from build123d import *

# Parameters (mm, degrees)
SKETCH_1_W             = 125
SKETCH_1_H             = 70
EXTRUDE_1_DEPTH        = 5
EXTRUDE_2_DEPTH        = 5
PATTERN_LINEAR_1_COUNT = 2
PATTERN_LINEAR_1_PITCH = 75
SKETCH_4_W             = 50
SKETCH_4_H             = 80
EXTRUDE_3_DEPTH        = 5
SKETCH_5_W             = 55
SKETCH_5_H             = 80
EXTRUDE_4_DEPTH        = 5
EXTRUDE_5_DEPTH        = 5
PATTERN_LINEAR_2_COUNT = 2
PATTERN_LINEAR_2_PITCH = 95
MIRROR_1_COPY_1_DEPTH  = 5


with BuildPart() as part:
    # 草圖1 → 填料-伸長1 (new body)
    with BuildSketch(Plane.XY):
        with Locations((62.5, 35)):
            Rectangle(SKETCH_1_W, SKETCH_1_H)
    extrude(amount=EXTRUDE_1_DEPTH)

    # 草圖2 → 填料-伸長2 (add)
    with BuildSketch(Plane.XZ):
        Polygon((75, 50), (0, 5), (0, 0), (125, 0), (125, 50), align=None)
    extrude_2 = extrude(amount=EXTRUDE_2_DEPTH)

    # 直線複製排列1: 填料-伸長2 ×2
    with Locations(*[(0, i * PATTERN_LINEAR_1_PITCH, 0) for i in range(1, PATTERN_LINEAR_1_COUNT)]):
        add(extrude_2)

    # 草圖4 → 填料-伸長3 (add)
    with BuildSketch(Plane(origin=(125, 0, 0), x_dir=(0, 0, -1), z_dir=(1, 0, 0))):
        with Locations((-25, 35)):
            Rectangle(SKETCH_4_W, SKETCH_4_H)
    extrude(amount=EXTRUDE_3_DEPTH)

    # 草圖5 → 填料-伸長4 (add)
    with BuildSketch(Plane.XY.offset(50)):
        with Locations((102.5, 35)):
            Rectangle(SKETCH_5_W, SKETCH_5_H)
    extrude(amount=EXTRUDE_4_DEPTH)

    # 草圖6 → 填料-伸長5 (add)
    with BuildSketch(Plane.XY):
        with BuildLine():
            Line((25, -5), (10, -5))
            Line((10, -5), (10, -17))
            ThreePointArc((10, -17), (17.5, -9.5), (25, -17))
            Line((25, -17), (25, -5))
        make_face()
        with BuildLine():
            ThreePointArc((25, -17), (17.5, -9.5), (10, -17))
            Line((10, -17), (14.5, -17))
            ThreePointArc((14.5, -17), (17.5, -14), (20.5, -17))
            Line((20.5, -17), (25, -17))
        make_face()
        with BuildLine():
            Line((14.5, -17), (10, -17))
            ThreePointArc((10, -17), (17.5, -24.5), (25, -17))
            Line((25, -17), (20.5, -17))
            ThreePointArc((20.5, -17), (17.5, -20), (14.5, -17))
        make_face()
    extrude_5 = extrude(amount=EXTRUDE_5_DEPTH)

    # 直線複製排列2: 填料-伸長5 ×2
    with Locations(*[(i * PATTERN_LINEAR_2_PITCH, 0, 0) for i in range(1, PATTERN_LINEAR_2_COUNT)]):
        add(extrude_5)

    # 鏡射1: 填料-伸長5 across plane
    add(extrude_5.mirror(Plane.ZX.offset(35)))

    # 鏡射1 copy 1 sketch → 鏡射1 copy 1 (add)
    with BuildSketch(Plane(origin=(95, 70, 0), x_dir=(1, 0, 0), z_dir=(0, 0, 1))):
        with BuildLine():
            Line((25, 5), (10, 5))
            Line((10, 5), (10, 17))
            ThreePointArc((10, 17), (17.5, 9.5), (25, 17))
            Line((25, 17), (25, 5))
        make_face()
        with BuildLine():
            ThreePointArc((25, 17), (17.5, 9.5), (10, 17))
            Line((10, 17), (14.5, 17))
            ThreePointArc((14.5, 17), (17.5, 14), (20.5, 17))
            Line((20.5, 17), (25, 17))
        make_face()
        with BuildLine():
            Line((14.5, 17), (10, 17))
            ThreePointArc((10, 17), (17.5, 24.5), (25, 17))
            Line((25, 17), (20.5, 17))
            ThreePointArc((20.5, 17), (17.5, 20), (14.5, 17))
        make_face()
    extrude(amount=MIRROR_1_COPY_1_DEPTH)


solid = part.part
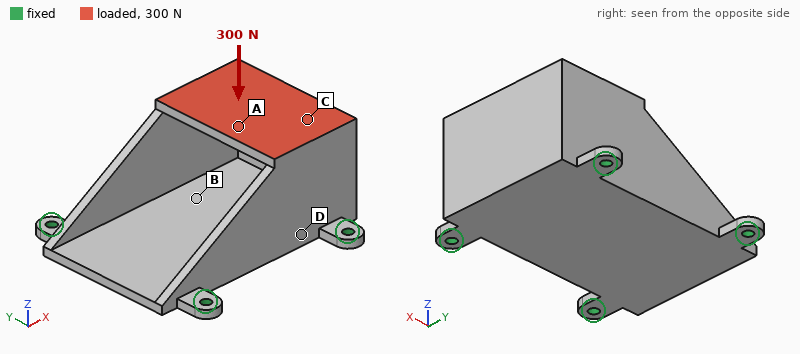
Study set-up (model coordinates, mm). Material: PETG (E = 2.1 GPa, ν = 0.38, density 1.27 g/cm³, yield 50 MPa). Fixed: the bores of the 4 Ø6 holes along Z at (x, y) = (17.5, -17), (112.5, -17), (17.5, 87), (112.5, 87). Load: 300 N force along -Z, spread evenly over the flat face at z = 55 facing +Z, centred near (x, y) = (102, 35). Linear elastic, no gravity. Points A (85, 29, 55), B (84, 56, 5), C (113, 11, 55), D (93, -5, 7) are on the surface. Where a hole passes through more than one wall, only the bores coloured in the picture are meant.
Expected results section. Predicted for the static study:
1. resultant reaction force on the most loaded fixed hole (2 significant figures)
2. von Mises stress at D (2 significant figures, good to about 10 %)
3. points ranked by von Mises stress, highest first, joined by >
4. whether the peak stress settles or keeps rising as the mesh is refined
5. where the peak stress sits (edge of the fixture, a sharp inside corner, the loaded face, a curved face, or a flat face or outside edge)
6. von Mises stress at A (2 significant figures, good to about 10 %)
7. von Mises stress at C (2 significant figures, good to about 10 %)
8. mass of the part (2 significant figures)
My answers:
140 N
1.0 MPa
A > C > D > B
keeps rising
edge of the fixture
3.5 MPa
2.1 MPa
170 g
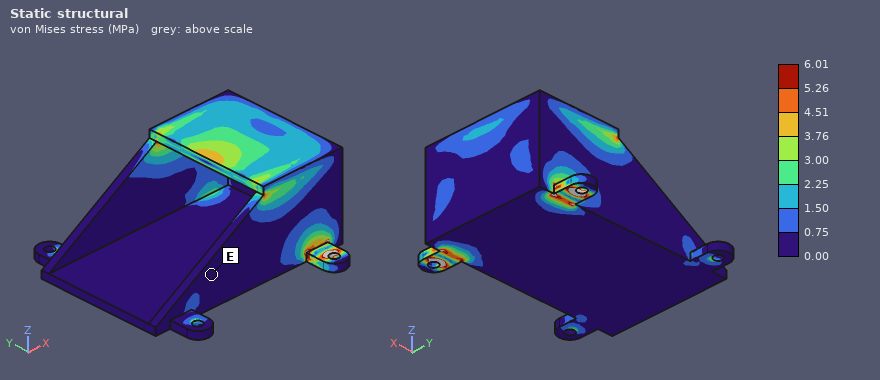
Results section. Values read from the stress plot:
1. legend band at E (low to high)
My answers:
0.00 to 0.75 MPa
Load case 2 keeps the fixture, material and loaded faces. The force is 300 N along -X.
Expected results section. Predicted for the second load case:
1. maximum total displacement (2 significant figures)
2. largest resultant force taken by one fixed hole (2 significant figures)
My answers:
0.28 mm
120 N
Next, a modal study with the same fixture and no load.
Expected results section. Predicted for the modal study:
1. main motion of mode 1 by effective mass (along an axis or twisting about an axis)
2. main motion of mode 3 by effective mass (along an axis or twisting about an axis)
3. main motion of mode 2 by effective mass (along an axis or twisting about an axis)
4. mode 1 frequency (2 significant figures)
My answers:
along Z
along Z
along Y
510 Hz
